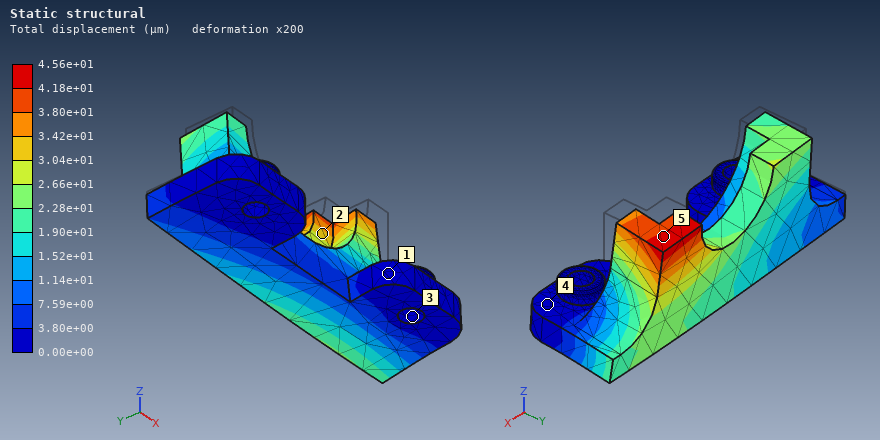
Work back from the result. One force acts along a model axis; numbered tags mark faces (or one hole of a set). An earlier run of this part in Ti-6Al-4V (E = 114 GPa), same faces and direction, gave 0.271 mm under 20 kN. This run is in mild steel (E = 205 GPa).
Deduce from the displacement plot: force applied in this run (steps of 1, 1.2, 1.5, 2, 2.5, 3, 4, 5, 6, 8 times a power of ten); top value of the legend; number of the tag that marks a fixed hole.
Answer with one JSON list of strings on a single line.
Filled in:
["6 kN", "4.56e+01 µm", "3"]
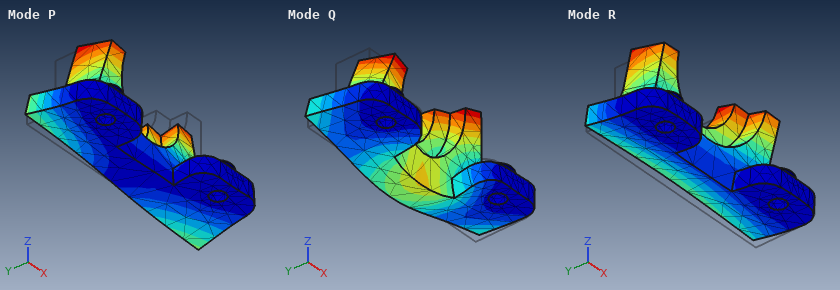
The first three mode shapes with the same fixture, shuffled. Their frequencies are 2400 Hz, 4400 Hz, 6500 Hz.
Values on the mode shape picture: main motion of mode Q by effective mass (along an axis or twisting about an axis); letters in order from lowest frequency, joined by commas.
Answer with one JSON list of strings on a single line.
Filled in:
["along Z", "R, P, Q"]
